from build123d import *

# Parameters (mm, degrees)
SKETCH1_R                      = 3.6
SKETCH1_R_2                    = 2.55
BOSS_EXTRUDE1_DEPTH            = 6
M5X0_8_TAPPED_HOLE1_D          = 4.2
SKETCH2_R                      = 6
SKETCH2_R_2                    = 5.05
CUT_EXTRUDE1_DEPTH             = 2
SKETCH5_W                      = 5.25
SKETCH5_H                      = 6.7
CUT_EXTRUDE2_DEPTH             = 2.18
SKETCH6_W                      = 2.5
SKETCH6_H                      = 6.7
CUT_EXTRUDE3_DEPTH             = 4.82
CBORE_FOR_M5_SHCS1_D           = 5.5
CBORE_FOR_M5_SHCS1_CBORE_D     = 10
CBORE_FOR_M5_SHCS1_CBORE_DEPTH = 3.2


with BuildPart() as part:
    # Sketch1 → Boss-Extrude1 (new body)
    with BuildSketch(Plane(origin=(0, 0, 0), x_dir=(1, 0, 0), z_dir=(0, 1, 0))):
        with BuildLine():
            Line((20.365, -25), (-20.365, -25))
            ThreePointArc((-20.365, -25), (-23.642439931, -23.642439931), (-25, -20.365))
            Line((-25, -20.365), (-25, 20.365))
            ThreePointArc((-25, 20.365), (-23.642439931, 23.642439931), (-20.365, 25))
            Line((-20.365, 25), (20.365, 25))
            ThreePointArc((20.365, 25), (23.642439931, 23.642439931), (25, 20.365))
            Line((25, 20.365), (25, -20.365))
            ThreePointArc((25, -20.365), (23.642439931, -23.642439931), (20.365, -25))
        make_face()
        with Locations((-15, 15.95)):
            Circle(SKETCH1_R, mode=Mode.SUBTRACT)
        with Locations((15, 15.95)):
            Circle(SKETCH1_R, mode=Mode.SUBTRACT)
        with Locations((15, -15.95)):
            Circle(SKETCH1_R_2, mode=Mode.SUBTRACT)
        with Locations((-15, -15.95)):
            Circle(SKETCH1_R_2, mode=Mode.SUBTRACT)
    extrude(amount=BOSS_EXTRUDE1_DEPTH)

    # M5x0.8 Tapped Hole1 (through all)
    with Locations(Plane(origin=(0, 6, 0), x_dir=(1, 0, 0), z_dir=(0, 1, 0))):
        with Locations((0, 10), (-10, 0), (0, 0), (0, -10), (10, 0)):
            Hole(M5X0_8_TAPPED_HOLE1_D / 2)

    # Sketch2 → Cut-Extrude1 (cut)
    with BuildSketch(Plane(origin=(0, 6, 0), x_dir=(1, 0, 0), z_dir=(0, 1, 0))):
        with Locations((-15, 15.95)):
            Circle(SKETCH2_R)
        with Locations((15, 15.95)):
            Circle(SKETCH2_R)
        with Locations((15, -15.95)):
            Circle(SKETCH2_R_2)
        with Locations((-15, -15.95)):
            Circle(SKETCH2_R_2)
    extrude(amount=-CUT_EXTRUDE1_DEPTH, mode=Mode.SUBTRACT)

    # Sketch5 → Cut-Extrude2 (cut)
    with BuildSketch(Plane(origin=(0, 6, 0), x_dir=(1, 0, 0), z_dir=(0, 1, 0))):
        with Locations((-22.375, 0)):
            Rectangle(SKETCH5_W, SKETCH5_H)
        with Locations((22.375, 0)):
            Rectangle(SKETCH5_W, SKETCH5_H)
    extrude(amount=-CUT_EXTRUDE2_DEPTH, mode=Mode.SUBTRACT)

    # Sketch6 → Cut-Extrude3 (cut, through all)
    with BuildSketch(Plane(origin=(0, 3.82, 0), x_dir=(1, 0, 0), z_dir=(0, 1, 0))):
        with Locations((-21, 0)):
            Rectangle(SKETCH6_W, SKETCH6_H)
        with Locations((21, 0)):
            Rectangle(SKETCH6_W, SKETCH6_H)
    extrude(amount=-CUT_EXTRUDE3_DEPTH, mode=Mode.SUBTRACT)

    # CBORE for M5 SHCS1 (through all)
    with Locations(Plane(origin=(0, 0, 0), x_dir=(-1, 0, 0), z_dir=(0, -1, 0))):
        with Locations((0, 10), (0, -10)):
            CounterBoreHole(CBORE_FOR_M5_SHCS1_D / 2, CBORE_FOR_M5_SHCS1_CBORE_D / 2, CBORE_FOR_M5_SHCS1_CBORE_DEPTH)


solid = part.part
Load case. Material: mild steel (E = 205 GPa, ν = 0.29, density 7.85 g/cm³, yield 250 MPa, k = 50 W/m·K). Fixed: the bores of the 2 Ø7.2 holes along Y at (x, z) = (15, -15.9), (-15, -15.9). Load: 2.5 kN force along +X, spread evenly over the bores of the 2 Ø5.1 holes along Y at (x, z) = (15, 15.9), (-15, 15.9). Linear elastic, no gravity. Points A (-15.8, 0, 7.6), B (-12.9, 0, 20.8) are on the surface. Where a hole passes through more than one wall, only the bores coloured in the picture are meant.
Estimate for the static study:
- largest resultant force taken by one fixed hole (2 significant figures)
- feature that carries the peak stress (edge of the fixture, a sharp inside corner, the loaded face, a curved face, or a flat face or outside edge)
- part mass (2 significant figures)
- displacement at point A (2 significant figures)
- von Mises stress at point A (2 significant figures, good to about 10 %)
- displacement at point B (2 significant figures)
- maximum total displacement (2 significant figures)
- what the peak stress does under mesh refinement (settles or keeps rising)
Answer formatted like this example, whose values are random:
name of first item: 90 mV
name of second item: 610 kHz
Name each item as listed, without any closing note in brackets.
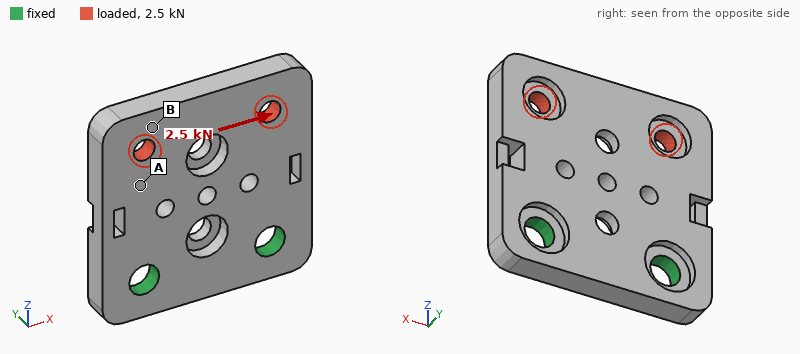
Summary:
largest resultant force taken by one fixed hole: 2.5 kN
feature that carries the peak stress: edge of the fixture
part mass: 98 g
displacement at point A: 9.2 µm
von Mises stress at point A: 27 MPa
displacement at point B: 14 µm
maximum total displacement: 18 µm
what the peak stress does under mesh refinement: keeps rising
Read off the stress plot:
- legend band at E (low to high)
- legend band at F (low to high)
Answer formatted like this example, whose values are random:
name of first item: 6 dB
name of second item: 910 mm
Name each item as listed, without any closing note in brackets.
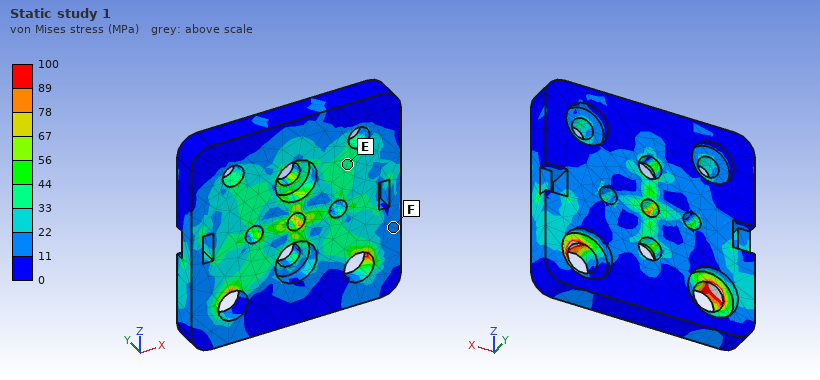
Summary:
legend band at E: 33 to 44 MPa
legend band at F: 11 to 22 MPa
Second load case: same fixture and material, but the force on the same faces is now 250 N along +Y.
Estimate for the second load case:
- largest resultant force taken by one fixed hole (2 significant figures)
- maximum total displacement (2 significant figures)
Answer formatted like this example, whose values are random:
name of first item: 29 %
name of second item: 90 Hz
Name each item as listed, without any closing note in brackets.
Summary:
largest resultant force taken by one fixed hole: 130 N
maximum total displacement: 32 µm
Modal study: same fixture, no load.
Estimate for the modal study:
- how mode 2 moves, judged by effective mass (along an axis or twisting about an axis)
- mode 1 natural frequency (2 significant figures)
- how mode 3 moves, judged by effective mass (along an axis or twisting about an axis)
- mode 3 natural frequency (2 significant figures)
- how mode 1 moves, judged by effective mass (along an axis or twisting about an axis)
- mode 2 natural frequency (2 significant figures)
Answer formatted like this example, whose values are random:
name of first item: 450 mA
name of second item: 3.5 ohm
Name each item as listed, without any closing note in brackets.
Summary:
how mode 2 moves, judged by effective mass: twisting about Z
mode 1 natural frequency: 2500 Hz
how mode 3 moves, judged by effective mass: along X
mode 3 natural frequency: 12 kHz
how mode 1 moves, judged by effective mass: along Y
mode 2 natural frequency: 5300 Hz
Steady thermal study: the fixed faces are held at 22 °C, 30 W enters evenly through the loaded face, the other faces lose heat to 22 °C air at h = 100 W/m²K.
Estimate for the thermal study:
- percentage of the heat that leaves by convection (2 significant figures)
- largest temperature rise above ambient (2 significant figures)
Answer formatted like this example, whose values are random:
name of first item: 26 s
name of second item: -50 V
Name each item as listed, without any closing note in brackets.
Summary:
percentage of the heat that leaves by convection: 52 %
largest temperature rise above ambient: 60 K
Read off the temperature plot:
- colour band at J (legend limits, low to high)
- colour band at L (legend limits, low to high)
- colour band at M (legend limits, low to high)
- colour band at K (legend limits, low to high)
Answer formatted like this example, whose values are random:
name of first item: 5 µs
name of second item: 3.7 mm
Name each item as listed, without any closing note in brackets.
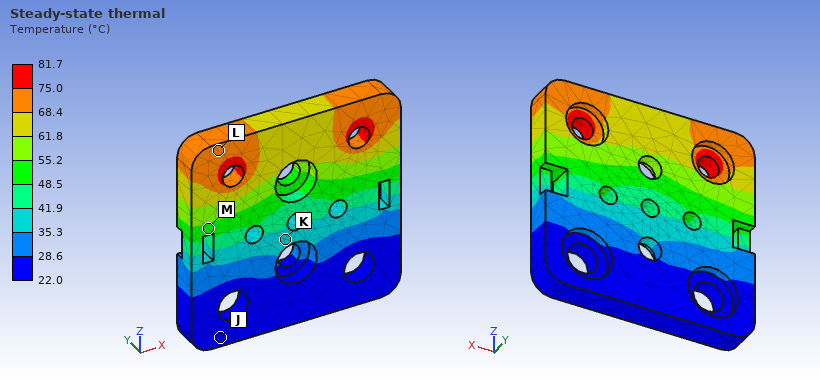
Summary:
colour band at J: 22.0 to 28.6 °C
colour band at L: 68.4 to 75.0 °C
colour band at M: 48.5 to 55.2 °C
colour band at K: 35.3 to 41.9 °C
